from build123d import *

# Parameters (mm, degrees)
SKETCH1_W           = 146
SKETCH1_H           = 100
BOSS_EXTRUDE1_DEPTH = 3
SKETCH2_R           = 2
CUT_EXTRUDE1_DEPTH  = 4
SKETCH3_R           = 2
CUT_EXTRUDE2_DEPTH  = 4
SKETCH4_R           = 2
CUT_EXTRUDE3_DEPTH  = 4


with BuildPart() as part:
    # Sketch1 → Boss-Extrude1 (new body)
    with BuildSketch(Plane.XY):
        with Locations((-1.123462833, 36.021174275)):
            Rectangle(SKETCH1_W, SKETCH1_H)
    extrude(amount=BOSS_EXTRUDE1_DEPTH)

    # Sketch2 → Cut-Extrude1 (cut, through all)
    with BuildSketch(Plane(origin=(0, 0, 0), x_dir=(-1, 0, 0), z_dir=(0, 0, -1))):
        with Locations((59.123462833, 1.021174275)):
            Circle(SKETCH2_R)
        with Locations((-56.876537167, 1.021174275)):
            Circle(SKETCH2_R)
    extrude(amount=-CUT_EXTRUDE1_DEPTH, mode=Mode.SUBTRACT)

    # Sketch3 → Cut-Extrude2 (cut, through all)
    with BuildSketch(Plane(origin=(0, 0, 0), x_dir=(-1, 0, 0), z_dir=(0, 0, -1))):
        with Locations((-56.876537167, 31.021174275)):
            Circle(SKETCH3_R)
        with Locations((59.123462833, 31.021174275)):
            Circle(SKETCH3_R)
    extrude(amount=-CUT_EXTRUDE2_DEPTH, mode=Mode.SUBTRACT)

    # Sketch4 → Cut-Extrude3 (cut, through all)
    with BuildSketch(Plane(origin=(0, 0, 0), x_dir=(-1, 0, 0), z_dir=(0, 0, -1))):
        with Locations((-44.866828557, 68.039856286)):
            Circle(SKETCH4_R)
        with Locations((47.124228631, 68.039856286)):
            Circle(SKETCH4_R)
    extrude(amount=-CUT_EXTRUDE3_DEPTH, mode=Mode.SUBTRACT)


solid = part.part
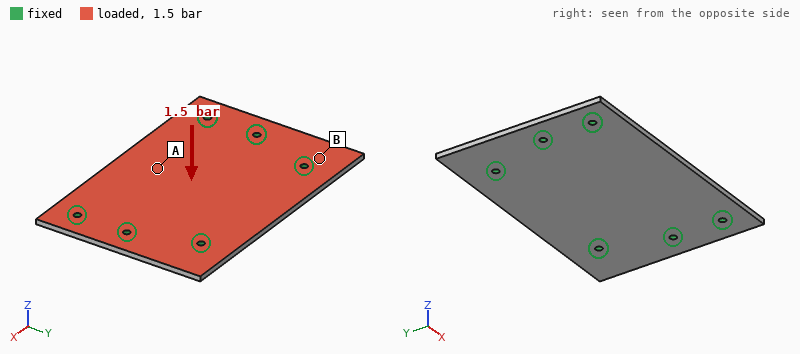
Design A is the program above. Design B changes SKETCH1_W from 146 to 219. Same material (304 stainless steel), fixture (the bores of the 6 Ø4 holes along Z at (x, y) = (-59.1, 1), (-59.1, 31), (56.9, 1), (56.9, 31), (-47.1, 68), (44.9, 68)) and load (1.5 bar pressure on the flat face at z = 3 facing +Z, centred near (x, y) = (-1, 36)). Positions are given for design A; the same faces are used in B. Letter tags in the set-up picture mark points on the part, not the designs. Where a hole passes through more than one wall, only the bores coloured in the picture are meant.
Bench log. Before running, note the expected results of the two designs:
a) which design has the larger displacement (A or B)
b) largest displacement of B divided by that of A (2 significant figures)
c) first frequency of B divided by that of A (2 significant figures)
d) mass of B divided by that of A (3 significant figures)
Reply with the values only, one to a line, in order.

B
2.6
0.62
1.50
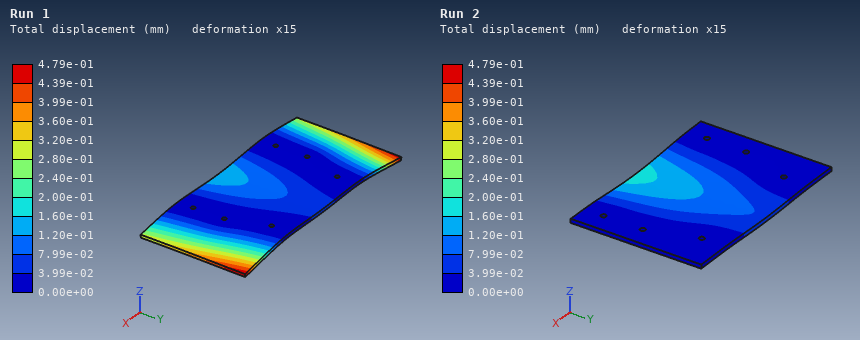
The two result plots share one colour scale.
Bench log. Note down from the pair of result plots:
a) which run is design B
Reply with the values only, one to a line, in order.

Run 1
